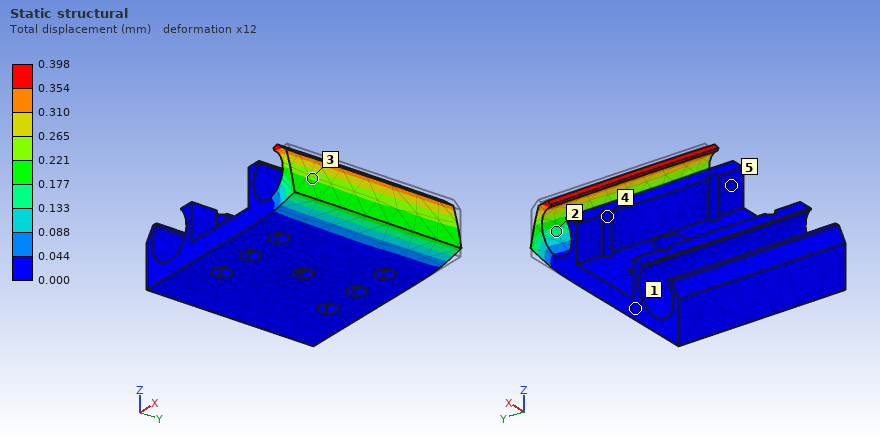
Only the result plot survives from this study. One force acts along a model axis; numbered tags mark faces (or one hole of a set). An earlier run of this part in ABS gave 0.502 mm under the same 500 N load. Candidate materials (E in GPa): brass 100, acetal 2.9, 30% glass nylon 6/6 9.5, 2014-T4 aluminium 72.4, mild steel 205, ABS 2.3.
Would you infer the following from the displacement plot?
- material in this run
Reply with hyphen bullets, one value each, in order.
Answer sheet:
- acetal
